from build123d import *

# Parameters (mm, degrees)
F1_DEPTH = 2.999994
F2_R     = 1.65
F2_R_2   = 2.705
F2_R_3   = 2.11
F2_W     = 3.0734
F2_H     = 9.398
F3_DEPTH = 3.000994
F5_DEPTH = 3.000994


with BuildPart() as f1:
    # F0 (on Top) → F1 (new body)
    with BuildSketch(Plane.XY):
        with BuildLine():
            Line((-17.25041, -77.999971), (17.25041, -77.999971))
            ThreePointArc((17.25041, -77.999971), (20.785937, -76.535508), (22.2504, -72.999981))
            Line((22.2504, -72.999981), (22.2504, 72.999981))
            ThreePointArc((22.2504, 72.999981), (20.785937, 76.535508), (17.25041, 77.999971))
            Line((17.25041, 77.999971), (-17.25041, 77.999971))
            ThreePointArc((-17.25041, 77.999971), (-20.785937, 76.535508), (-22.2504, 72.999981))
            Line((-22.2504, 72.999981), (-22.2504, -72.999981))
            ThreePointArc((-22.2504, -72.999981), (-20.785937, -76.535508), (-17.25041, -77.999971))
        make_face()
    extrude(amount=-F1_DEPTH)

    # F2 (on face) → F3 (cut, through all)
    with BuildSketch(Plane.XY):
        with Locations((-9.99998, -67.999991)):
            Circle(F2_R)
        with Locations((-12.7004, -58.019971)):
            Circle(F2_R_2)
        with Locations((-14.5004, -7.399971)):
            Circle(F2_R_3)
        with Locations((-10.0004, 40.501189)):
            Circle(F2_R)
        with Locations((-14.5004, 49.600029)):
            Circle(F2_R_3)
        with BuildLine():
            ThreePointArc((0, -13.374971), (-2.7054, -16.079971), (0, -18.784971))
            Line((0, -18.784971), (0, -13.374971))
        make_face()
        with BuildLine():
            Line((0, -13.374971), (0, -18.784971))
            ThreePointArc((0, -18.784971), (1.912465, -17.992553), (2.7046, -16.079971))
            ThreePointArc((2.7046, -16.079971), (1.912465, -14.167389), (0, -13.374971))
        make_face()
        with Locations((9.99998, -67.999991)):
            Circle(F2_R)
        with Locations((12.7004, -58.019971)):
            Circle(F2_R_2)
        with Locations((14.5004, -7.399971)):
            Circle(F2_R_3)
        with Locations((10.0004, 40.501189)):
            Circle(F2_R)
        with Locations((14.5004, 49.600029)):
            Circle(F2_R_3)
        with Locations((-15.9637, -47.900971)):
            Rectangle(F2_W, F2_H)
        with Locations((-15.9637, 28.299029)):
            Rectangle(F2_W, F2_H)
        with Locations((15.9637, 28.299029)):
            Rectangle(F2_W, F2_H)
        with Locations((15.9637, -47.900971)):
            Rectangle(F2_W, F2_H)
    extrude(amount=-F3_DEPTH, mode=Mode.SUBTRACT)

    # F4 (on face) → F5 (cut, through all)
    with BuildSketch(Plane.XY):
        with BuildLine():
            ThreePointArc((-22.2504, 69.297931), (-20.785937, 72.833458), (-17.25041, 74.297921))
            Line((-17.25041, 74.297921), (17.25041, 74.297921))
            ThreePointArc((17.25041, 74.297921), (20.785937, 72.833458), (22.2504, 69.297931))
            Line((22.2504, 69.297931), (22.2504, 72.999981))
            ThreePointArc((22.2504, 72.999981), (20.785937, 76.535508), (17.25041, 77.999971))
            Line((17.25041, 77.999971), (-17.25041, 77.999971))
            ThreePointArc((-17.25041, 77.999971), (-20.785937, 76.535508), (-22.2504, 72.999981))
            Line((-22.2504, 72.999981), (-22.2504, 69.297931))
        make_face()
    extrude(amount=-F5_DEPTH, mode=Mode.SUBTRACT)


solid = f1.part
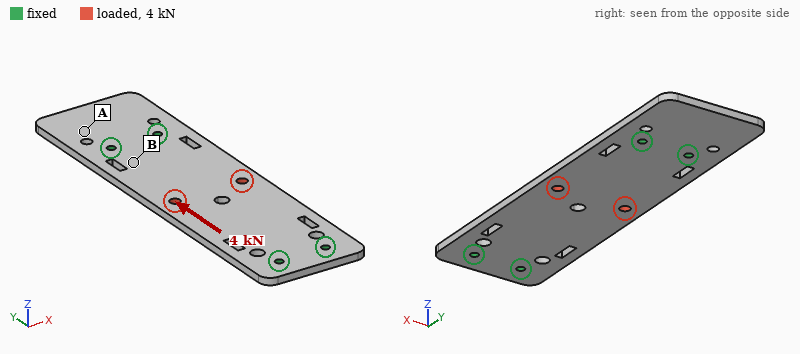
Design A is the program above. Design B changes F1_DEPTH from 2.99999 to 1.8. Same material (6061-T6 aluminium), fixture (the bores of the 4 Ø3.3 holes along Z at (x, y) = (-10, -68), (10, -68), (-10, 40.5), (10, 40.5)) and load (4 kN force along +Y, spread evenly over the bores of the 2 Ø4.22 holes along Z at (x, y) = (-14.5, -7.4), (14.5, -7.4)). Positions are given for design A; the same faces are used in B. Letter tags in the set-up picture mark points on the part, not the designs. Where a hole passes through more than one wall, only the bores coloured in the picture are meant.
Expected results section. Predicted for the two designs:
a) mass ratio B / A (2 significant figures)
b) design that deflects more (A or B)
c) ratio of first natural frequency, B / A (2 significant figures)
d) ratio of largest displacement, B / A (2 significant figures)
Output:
0.60
B
0.61
1.7
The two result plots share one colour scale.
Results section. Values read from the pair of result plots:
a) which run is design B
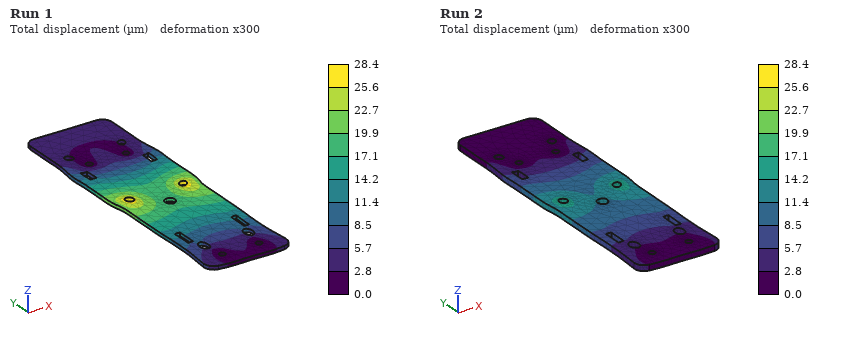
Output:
Run 1
